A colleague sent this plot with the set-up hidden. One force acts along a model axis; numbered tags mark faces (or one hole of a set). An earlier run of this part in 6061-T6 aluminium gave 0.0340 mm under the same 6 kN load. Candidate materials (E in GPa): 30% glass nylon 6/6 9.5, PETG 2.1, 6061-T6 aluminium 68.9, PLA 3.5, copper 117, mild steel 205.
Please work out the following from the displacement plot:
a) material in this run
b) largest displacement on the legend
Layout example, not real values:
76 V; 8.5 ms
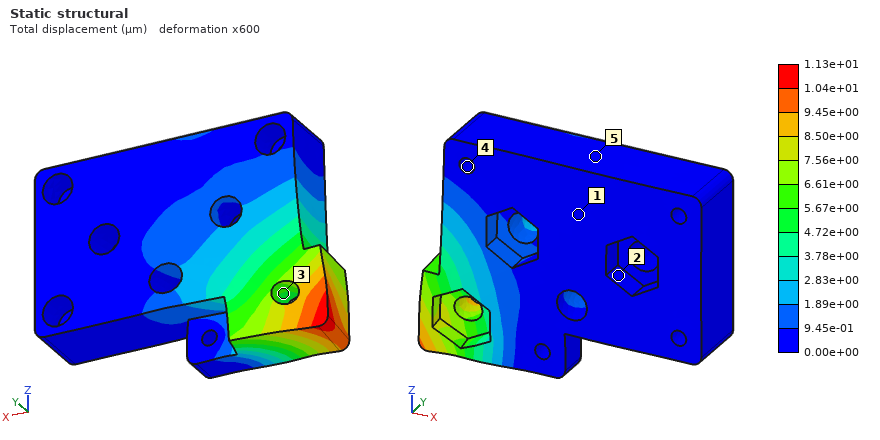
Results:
mild steel; 1.13e+01 µm
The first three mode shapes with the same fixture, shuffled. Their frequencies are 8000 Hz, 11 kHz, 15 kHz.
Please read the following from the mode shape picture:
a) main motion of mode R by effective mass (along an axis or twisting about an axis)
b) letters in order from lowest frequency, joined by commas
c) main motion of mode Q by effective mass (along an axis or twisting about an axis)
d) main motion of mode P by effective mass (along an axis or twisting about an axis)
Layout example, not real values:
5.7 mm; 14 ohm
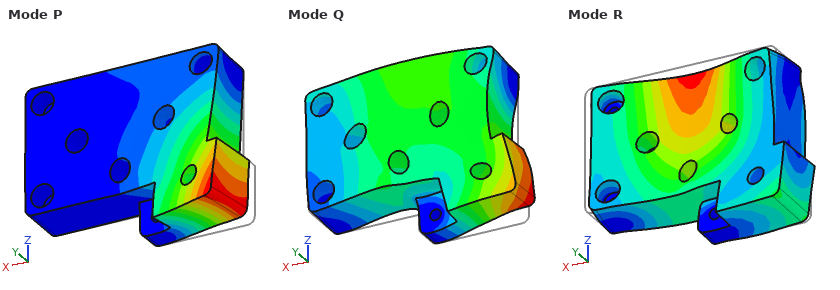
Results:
along Y; P, R, Q; along Z; along Y
